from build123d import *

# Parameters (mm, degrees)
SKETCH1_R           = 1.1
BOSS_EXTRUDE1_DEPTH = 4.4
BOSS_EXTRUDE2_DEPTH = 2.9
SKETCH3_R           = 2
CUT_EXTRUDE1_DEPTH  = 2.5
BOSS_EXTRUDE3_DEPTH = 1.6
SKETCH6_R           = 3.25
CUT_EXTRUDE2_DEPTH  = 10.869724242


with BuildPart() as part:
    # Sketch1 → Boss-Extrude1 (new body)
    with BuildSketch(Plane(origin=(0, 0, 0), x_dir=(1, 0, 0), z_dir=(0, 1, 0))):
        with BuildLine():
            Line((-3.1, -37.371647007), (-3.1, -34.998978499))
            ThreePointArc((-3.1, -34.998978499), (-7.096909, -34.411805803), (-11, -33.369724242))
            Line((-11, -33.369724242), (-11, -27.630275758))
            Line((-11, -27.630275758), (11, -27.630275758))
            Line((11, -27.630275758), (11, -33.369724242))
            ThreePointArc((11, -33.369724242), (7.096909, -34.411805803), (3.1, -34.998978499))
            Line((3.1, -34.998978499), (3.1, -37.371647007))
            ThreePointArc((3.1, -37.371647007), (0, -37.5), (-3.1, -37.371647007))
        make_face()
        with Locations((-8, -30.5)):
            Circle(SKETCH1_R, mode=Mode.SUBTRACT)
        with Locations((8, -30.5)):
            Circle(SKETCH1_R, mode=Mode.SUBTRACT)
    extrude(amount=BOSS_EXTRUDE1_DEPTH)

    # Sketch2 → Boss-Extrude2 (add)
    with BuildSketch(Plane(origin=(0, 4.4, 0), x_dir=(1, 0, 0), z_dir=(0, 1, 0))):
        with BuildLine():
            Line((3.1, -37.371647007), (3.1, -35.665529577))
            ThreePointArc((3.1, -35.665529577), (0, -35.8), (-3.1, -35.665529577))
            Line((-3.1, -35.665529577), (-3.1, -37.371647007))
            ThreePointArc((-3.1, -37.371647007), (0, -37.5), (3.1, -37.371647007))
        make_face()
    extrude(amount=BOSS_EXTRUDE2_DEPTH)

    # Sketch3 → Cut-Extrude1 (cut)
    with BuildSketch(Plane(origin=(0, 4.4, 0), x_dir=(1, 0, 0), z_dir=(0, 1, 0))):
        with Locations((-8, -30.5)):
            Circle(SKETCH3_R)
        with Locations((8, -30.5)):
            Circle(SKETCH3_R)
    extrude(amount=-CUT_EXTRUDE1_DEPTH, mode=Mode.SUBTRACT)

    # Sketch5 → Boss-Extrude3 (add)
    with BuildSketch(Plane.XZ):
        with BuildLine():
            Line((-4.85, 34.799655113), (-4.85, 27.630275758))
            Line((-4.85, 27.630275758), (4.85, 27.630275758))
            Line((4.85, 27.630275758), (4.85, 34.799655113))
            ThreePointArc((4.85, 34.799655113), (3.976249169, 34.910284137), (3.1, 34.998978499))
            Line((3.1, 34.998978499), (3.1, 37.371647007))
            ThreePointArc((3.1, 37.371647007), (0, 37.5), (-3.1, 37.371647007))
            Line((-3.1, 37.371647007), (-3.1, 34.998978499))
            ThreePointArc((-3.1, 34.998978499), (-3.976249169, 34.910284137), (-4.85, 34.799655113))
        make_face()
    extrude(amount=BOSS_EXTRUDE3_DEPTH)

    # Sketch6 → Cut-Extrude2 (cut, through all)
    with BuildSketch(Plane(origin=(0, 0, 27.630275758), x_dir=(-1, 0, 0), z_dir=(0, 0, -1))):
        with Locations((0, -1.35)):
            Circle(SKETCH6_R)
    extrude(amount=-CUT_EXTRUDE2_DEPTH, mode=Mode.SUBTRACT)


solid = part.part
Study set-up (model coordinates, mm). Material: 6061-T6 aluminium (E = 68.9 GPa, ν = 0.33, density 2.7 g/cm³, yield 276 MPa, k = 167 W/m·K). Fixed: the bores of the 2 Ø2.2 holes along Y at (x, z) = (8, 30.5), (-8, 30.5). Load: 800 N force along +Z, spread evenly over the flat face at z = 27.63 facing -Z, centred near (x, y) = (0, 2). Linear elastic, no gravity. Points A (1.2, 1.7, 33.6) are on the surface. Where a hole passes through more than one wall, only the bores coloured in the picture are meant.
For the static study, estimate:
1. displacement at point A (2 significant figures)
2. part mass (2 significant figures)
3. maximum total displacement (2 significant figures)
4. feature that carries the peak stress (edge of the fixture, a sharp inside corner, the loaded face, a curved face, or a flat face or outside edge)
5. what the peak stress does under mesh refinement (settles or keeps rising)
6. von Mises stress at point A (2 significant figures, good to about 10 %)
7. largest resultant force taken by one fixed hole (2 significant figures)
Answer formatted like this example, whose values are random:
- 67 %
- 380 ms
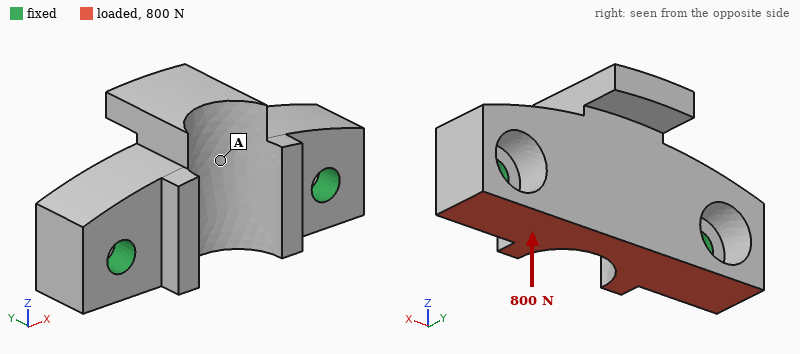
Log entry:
- 5.7 µm
- 1.7 g
- 14 µm
- edge of the fixture
- keeps rising
- 20 MPa
- 400 N
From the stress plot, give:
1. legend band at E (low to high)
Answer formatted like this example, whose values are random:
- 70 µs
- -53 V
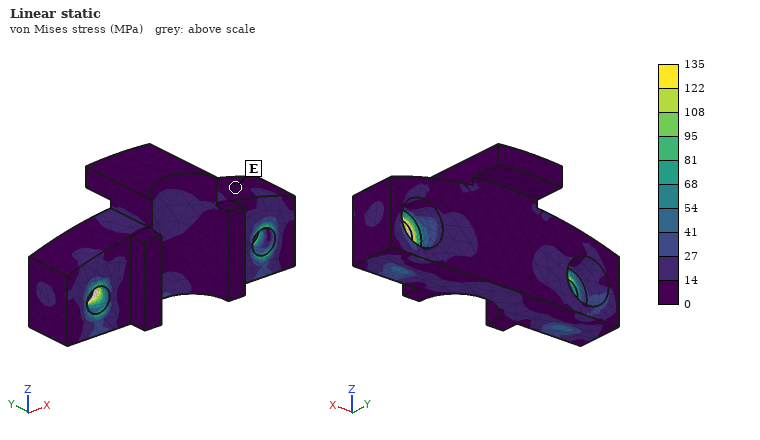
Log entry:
- 0 to 14 MPa
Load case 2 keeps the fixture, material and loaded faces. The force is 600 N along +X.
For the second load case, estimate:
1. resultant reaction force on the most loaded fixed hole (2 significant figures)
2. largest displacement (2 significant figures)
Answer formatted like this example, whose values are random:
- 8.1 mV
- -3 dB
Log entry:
- 310 N
- 3.7 µm
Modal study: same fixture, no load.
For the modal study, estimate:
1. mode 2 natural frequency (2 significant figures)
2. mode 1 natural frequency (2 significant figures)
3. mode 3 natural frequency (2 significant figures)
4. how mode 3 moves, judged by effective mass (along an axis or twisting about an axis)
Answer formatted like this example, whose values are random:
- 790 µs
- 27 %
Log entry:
- 48 kHz
- 25 kHz
- 60 kHz
- along Z
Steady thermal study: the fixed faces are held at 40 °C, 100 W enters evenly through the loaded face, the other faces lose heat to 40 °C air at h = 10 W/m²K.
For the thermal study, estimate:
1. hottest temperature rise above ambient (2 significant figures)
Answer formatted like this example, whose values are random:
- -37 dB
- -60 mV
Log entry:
- 58 K
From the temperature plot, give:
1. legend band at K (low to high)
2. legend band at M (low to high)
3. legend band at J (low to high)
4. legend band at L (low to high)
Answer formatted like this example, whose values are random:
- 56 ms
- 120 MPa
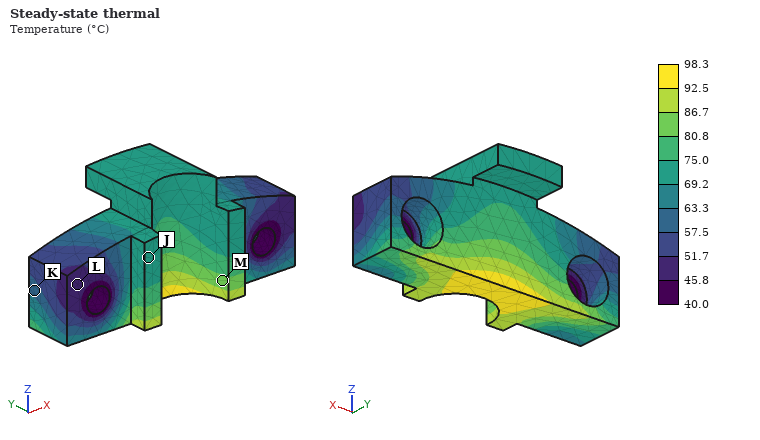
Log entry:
- 57.5 to 63.3 °C
- 80.8 to 86.7 °C
- 69.2 to 75.0 °C
- 45.8 to 51.7 °C
